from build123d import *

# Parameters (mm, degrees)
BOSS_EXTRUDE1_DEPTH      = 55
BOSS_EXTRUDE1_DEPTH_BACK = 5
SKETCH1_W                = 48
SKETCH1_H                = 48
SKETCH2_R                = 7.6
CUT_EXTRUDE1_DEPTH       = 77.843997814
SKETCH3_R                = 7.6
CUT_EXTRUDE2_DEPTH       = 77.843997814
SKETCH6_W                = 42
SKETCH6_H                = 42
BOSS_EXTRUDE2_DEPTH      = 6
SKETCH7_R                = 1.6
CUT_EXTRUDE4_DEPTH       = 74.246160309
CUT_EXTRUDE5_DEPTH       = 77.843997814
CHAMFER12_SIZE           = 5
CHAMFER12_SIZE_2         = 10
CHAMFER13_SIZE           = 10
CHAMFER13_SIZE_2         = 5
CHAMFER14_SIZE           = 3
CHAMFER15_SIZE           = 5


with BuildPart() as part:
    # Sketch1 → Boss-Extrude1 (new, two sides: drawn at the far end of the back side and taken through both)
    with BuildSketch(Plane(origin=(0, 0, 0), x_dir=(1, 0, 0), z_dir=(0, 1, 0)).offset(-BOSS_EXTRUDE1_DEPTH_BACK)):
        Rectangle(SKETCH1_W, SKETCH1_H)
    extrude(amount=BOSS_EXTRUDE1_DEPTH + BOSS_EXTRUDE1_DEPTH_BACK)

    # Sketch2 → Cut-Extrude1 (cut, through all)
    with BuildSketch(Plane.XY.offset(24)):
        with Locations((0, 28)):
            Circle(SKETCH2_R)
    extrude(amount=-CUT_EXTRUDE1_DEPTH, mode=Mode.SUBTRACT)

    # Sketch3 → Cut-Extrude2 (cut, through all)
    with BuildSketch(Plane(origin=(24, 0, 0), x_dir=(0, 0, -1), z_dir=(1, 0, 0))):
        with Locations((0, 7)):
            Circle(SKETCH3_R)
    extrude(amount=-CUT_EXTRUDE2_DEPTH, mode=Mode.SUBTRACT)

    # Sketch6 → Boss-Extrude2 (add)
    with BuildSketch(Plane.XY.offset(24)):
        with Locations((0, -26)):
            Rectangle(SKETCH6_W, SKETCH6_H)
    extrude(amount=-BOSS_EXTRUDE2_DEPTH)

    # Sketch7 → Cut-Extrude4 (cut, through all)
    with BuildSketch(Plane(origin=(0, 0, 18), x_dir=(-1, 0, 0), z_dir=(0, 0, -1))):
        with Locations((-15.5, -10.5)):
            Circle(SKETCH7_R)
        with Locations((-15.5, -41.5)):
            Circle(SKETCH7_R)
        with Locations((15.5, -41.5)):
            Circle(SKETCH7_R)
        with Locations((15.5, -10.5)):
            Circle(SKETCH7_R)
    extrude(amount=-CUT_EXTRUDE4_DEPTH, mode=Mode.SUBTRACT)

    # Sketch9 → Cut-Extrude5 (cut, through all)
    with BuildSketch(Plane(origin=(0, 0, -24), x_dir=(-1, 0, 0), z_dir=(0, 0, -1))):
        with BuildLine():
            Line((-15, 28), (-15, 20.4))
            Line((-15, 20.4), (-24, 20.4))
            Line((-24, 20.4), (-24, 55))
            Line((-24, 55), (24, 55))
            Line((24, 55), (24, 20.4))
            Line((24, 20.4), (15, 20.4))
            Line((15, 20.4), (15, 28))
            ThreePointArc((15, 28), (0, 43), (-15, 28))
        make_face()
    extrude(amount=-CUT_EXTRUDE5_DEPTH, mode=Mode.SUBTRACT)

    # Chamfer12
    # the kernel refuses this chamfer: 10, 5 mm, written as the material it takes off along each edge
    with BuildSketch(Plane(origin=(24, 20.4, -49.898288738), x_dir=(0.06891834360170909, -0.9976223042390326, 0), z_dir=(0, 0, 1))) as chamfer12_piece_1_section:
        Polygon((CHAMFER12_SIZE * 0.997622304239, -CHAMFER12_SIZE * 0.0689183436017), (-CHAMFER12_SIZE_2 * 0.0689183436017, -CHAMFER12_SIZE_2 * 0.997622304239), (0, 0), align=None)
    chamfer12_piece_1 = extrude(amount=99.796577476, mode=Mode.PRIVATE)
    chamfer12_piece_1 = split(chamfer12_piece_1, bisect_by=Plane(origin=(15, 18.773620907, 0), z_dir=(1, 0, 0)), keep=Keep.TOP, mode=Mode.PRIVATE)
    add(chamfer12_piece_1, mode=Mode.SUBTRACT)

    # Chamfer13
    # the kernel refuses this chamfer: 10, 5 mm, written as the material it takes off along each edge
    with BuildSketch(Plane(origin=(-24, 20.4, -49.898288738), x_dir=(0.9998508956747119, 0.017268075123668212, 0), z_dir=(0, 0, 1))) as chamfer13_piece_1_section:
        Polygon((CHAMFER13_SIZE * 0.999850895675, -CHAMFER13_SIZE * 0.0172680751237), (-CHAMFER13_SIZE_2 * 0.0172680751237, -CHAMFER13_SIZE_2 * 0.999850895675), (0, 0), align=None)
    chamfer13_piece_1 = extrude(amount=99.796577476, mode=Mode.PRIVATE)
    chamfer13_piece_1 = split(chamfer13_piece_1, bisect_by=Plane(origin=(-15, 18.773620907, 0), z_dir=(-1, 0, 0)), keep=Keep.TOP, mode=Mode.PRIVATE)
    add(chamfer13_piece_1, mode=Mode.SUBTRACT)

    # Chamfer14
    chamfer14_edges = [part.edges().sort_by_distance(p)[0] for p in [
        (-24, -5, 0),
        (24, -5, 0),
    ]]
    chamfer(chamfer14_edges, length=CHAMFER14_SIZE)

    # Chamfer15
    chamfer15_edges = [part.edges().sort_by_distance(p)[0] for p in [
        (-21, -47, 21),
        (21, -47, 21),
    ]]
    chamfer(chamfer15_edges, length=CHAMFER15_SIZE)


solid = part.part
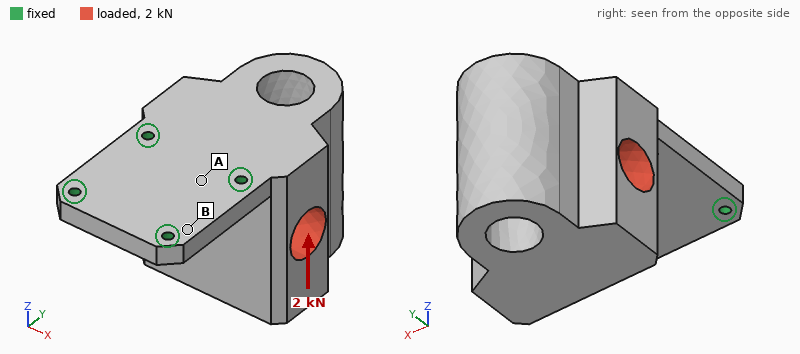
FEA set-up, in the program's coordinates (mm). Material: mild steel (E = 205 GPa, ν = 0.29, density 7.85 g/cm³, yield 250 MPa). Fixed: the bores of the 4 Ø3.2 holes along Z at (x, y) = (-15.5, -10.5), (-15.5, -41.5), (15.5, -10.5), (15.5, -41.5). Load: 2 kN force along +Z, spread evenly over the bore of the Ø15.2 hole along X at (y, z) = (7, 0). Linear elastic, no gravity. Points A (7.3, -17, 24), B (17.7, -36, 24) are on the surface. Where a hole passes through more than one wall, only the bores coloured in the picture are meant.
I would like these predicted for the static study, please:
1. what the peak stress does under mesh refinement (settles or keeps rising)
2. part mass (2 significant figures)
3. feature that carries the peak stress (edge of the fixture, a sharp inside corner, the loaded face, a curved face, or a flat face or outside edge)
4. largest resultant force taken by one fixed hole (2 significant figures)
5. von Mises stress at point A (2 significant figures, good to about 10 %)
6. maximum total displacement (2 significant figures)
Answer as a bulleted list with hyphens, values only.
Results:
- keeps rising
- 600 g
- edge of the fixture
- 1.2 kN
- 28 MPa
- 0.12 mm
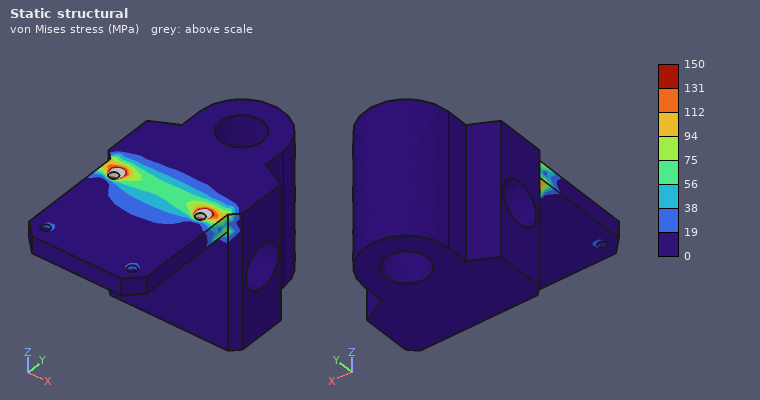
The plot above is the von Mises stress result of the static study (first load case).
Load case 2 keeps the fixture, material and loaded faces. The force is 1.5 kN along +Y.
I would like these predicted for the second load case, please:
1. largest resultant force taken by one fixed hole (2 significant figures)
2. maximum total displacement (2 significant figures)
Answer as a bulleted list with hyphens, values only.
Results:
- 650 N
- 0.13 mm
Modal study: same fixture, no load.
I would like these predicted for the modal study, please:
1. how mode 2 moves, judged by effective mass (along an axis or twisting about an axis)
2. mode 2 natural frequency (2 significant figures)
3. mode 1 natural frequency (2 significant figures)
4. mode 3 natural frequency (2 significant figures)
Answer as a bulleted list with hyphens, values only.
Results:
- along X
- 3000 Hz
- 770 Hz
- 5800 Hz
